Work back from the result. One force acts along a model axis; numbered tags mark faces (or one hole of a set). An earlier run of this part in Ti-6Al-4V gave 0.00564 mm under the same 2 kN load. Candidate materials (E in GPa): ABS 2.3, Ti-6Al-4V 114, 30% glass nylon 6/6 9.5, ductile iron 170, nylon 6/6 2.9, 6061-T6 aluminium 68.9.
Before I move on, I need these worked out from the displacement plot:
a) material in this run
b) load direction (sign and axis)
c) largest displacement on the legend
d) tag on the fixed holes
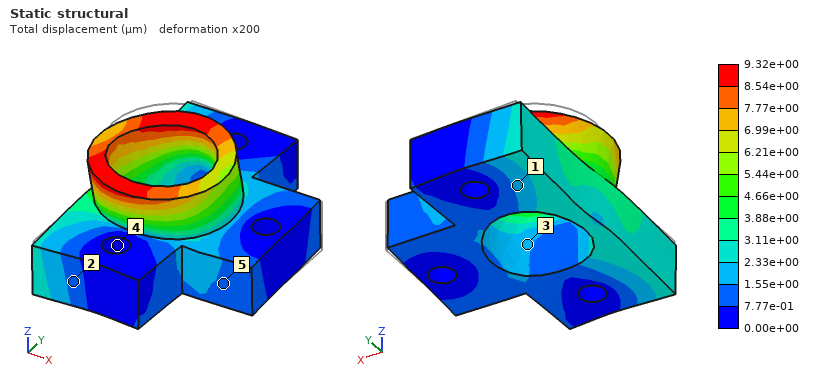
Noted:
6061-T6 aluminium
-Y
9.32e+00 µm
4
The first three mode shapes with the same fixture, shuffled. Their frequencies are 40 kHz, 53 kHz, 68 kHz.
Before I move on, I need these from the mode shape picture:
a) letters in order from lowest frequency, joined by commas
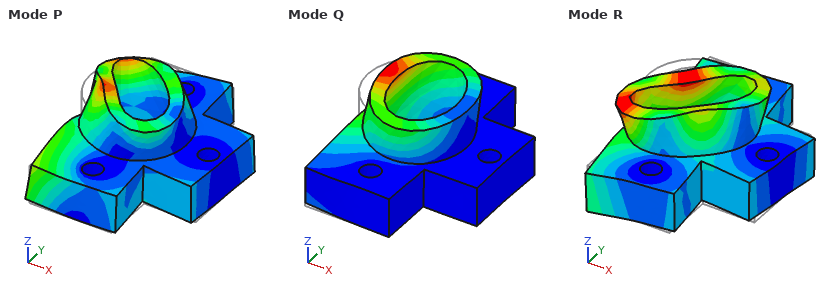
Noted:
Q, R, P
